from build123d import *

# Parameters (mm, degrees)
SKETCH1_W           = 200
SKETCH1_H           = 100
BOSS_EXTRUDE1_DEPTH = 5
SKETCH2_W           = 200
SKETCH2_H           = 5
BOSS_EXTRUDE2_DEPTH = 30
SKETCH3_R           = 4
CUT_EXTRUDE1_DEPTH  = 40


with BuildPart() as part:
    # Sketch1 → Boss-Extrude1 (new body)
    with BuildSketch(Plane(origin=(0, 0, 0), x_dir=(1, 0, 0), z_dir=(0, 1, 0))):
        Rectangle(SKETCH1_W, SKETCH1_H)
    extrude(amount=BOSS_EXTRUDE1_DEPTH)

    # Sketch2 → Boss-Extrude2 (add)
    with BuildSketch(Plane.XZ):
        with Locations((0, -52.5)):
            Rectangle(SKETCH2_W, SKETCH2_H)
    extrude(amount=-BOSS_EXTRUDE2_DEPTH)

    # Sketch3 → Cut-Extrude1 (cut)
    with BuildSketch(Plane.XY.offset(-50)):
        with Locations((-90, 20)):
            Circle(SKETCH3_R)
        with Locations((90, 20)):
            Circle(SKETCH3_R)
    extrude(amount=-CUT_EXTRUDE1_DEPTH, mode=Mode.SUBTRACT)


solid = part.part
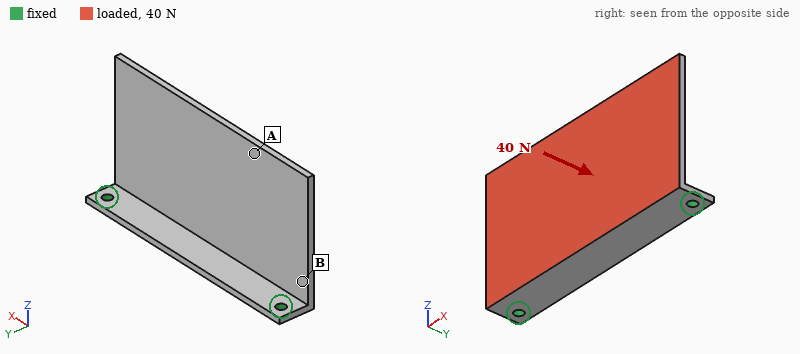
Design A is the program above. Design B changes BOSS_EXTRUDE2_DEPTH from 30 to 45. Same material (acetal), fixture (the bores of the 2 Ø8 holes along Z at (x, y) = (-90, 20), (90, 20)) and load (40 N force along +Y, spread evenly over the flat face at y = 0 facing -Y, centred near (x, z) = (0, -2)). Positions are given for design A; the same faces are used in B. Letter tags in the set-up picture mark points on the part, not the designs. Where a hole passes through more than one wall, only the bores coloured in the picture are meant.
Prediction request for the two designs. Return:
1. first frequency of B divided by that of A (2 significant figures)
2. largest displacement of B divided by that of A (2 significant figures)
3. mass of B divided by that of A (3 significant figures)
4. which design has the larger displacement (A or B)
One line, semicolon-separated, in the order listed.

1.1; 0.86; 1.12; A
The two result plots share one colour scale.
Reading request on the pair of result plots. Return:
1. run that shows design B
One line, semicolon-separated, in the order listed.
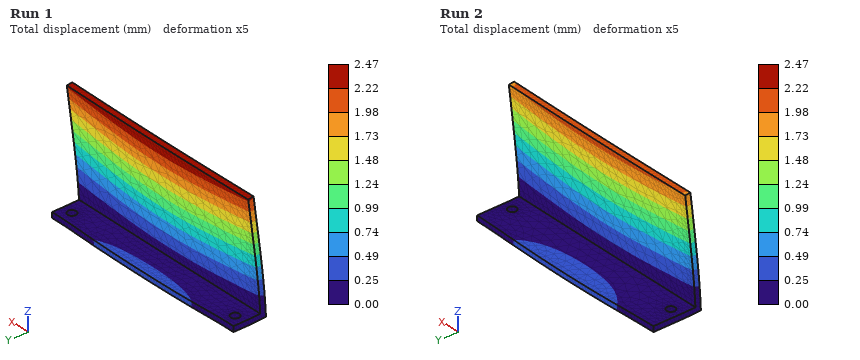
Run 2
